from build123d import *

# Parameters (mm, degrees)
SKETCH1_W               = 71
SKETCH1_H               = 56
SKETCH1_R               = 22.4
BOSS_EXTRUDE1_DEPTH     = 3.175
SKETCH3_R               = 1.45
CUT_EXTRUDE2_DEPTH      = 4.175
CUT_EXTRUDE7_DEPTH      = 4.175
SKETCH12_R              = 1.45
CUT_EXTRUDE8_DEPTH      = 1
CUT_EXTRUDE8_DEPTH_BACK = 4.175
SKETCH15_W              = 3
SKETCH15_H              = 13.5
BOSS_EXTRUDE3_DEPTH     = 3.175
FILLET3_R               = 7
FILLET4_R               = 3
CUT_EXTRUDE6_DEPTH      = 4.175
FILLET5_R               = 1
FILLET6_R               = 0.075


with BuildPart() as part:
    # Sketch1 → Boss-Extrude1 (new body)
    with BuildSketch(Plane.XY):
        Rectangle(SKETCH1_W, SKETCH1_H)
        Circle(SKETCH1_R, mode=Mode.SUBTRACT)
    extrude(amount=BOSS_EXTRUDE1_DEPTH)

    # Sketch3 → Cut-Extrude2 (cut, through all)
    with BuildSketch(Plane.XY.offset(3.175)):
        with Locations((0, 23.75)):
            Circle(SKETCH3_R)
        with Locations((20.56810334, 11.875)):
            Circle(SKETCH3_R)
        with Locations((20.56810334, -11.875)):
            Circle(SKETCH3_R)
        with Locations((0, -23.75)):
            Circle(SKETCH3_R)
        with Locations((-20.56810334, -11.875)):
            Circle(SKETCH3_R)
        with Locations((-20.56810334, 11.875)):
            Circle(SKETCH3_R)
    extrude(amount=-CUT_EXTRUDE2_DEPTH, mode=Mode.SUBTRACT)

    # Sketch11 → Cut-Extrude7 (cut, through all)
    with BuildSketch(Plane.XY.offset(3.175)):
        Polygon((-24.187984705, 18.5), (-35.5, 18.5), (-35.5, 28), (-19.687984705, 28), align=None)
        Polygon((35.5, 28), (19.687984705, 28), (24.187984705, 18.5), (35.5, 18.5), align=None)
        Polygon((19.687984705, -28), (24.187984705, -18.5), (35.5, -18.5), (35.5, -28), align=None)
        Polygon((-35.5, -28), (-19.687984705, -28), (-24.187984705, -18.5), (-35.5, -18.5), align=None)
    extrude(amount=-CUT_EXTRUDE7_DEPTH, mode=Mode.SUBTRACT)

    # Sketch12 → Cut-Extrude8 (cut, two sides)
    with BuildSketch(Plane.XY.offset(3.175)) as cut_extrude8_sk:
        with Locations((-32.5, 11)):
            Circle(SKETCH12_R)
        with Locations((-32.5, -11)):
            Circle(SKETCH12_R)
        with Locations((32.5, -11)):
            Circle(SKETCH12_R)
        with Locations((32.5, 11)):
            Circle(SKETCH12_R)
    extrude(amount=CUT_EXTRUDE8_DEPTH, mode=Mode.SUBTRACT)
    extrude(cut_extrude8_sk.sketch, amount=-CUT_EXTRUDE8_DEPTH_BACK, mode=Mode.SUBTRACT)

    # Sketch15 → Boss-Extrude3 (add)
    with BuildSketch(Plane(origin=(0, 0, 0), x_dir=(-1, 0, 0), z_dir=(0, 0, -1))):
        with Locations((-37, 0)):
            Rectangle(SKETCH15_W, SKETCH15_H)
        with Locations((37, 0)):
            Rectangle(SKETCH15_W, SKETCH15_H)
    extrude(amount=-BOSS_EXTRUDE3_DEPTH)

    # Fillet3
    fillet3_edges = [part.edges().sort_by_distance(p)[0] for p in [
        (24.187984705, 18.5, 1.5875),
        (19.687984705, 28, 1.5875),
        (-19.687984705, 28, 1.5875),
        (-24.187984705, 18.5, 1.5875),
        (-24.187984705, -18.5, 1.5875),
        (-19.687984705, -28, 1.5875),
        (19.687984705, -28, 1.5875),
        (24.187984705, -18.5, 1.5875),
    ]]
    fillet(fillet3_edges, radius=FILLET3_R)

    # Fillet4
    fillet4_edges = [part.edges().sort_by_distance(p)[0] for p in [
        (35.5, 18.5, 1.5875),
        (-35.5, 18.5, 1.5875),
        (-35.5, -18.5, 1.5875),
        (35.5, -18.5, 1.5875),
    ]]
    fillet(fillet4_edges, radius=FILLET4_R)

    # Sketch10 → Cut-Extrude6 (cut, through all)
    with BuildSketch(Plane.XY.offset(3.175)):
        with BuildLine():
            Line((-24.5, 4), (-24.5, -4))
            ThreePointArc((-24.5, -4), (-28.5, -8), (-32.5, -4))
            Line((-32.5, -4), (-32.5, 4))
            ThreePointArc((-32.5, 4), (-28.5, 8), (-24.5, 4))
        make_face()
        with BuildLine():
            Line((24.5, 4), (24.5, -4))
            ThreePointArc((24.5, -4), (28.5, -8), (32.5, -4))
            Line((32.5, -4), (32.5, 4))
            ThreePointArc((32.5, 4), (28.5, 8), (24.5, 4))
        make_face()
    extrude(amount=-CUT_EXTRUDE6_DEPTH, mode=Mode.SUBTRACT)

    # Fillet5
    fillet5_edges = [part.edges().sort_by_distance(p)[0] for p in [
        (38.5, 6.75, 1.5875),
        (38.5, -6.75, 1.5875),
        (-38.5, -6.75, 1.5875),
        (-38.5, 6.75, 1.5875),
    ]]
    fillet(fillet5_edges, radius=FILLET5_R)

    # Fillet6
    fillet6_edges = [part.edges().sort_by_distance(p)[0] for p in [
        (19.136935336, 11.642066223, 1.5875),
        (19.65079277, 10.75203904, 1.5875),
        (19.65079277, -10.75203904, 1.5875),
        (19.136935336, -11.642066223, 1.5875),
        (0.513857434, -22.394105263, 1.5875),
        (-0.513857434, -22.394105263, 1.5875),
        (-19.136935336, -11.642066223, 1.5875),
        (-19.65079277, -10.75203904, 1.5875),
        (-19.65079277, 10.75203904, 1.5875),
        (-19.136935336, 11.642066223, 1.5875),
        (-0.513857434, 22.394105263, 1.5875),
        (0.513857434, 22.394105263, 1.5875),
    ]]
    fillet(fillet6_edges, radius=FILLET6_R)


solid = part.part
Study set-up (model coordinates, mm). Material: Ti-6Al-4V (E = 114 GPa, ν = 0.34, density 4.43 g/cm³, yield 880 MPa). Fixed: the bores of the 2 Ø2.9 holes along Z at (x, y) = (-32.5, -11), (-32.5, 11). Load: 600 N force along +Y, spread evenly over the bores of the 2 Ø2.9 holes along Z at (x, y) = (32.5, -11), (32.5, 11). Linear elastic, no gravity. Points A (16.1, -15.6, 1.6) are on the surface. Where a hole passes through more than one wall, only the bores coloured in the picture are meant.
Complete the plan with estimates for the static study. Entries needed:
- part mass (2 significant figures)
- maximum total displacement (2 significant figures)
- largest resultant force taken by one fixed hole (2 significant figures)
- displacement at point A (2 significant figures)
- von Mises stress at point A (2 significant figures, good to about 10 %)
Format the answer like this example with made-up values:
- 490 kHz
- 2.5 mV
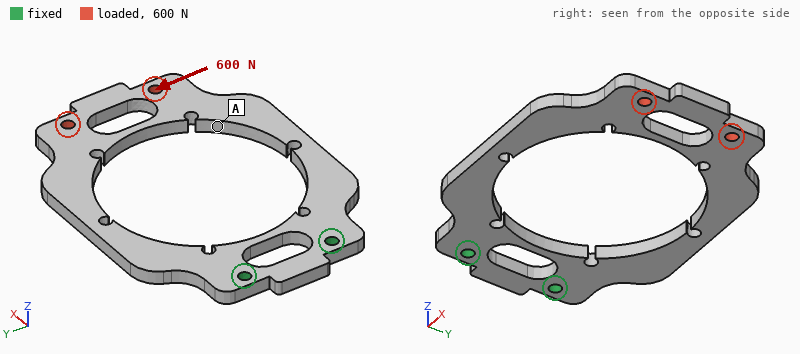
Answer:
- 23 g
- 0.65 mm
- 830 N
- 0.52 mm
- 85 MPa
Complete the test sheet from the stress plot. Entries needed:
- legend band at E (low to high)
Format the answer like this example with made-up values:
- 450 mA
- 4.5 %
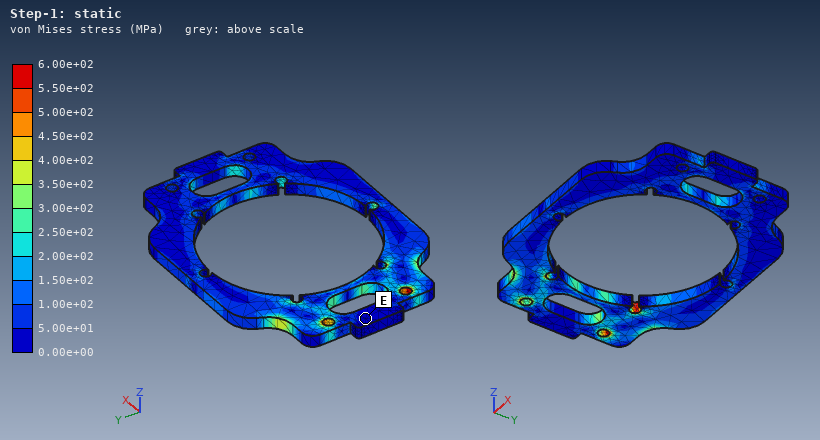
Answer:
- 0.00e+00 to 5.00e+01 MPa
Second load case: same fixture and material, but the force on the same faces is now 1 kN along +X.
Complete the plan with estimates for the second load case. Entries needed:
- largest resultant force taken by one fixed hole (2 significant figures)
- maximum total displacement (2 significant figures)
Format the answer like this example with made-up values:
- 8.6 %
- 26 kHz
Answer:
- 690 N
- 0.11 mm
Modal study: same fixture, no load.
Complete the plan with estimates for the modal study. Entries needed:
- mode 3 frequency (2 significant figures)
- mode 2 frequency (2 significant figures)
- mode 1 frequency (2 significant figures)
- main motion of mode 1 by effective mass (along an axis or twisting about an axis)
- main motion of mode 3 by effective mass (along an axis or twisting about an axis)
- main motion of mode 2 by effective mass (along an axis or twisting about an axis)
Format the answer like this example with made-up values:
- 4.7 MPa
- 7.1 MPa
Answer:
- 1600 Hz
- 1100 Hz
- 410 Hz
- along Z
- along Y
- twisting about X
